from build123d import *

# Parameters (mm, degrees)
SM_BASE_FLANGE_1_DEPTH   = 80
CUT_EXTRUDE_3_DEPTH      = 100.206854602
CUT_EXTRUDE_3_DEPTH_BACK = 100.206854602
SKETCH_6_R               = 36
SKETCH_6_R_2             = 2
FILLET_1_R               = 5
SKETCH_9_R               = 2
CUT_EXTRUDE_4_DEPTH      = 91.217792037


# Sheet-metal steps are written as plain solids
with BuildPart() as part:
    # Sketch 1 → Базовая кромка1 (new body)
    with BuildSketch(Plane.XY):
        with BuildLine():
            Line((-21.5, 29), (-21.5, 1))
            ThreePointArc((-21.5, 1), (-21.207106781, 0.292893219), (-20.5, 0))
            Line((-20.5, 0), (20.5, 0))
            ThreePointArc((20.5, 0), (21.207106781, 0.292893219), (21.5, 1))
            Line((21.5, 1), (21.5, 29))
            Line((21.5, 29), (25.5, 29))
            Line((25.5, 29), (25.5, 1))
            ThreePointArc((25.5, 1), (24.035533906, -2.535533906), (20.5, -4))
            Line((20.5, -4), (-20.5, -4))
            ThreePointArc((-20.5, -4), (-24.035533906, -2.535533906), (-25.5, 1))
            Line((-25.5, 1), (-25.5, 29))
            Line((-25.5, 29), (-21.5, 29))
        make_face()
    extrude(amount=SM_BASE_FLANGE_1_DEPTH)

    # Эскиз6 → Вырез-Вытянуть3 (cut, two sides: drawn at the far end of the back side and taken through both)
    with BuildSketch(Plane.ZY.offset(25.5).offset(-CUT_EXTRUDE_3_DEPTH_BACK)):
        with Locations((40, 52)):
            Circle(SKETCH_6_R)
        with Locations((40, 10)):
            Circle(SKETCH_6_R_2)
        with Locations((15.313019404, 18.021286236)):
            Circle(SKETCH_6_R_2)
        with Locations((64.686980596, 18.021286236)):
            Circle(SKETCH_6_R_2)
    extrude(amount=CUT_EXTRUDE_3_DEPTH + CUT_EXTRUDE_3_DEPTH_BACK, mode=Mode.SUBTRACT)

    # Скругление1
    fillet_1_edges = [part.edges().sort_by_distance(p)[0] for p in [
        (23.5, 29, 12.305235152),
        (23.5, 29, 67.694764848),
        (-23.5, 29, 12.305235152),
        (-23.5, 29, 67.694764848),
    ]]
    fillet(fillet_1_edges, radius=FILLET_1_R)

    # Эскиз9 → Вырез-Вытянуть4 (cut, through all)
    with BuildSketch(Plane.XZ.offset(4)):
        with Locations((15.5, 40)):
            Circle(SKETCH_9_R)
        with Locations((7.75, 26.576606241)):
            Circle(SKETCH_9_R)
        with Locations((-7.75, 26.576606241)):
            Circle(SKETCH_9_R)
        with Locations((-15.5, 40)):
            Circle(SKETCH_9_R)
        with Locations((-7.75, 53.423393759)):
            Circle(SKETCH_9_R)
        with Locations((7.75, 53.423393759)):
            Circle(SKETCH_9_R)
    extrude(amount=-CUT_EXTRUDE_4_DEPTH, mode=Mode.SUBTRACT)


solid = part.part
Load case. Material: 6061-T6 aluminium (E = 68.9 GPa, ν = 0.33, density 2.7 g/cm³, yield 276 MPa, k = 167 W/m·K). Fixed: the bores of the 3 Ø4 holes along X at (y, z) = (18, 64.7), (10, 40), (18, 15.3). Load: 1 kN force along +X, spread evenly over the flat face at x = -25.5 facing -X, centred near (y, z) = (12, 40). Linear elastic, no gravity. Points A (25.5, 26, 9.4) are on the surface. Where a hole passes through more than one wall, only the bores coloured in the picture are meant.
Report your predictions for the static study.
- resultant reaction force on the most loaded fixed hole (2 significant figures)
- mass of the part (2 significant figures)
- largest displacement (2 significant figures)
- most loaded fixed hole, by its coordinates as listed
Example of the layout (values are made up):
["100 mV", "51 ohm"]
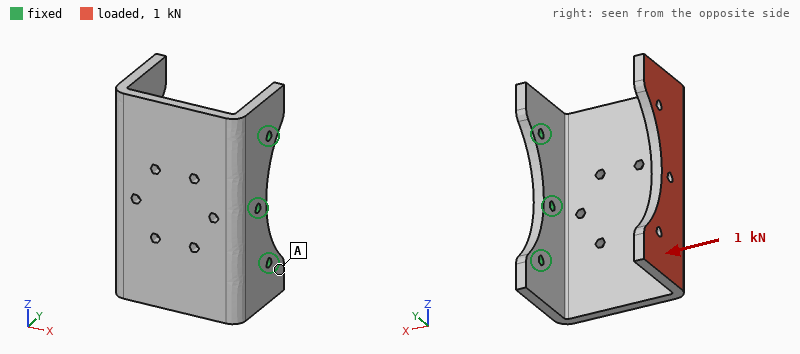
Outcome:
["410 N", "79 g", "1.1 mm", "(10, 40)"]
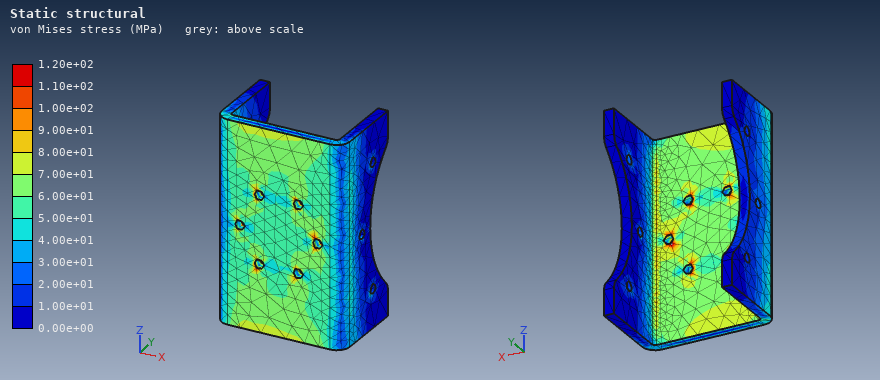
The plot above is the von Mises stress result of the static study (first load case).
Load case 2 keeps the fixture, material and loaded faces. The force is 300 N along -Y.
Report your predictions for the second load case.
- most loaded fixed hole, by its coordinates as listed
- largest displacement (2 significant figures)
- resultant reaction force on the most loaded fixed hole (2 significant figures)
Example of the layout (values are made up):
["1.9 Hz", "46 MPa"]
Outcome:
["(10, 40)", "0.88 mm", "460 N"]
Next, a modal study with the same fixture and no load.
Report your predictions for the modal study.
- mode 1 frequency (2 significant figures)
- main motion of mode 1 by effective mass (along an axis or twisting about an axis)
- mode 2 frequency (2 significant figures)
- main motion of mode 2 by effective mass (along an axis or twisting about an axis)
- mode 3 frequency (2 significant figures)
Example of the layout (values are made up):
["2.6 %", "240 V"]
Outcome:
["600 Hz", "along Y", "1000 Hz", "along Z", "1800 Hz"]
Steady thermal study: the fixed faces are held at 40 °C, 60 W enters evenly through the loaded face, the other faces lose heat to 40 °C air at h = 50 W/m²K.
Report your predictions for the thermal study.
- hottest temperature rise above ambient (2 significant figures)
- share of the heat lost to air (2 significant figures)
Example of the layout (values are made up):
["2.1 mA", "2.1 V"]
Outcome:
["69 K", "37 %"]
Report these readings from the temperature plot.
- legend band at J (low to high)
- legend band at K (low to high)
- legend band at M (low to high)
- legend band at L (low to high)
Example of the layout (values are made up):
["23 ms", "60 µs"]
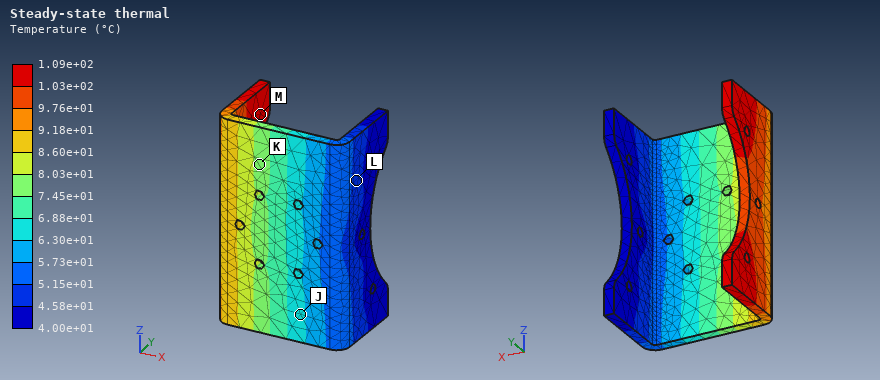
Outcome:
["6.30e+01 to 6.88e+01 °C", "7.45e+01 to 8.03e+01 °C", "1.03e+02 to 1.09e+02 °C", "4.58e+01 to 5.15e+01 °C"]
